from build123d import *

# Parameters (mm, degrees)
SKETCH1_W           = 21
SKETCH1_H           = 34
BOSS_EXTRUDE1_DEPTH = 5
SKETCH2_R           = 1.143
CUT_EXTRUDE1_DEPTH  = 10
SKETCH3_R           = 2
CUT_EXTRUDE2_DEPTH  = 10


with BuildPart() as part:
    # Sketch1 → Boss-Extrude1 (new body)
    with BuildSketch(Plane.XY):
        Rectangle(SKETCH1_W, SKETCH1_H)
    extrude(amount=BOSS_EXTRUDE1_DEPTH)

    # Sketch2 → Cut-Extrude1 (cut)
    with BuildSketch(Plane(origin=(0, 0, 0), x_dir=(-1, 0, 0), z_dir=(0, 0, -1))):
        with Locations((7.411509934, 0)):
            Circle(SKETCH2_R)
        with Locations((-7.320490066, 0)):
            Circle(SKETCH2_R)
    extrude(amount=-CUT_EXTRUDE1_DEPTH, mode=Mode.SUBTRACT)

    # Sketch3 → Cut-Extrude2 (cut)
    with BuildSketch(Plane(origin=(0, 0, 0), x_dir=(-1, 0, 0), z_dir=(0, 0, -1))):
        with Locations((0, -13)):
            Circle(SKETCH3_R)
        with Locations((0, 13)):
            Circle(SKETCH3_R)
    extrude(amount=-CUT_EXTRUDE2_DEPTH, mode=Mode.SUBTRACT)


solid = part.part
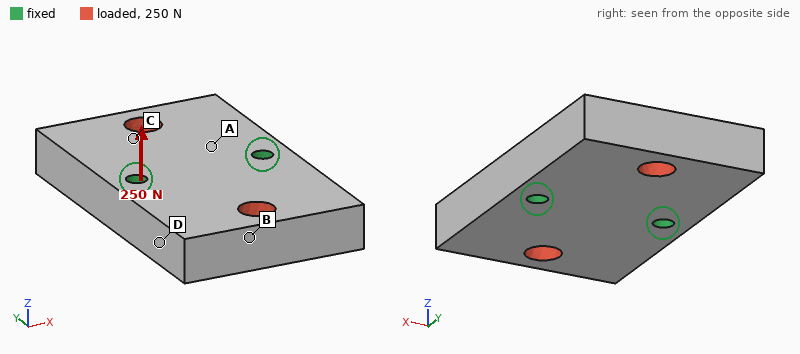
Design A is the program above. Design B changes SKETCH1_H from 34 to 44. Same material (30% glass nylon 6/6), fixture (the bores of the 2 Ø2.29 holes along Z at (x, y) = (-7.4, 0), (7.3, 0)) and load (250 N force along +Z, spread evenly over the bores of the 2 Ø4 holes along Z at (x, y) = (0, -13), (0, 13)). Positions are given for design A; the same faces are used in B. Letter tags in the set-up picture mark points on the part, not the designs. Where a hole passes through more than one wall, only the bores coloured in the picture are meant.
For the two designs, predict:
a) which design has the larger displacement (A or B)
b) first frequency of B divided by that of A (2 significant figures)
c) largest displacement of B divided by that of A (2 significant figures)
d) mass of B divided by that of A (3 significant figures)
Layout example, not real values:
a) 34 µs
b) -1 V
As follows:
a) B
b) 0.61
c) 1.3
d) 1.31
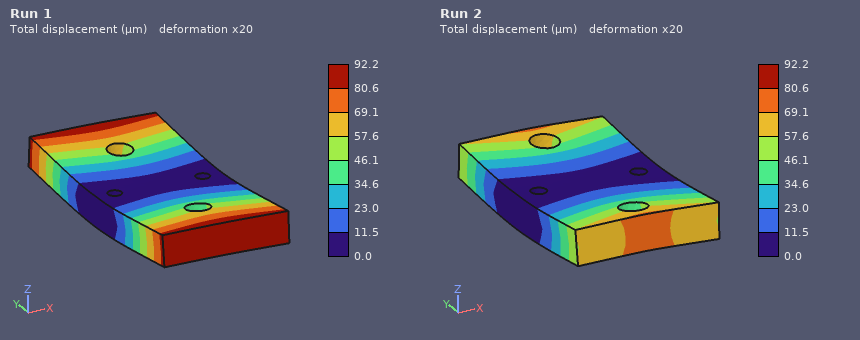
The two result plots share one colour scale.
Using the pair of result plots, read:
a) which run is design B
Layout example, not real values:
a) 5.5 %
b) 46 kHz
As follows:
a) Run 1
